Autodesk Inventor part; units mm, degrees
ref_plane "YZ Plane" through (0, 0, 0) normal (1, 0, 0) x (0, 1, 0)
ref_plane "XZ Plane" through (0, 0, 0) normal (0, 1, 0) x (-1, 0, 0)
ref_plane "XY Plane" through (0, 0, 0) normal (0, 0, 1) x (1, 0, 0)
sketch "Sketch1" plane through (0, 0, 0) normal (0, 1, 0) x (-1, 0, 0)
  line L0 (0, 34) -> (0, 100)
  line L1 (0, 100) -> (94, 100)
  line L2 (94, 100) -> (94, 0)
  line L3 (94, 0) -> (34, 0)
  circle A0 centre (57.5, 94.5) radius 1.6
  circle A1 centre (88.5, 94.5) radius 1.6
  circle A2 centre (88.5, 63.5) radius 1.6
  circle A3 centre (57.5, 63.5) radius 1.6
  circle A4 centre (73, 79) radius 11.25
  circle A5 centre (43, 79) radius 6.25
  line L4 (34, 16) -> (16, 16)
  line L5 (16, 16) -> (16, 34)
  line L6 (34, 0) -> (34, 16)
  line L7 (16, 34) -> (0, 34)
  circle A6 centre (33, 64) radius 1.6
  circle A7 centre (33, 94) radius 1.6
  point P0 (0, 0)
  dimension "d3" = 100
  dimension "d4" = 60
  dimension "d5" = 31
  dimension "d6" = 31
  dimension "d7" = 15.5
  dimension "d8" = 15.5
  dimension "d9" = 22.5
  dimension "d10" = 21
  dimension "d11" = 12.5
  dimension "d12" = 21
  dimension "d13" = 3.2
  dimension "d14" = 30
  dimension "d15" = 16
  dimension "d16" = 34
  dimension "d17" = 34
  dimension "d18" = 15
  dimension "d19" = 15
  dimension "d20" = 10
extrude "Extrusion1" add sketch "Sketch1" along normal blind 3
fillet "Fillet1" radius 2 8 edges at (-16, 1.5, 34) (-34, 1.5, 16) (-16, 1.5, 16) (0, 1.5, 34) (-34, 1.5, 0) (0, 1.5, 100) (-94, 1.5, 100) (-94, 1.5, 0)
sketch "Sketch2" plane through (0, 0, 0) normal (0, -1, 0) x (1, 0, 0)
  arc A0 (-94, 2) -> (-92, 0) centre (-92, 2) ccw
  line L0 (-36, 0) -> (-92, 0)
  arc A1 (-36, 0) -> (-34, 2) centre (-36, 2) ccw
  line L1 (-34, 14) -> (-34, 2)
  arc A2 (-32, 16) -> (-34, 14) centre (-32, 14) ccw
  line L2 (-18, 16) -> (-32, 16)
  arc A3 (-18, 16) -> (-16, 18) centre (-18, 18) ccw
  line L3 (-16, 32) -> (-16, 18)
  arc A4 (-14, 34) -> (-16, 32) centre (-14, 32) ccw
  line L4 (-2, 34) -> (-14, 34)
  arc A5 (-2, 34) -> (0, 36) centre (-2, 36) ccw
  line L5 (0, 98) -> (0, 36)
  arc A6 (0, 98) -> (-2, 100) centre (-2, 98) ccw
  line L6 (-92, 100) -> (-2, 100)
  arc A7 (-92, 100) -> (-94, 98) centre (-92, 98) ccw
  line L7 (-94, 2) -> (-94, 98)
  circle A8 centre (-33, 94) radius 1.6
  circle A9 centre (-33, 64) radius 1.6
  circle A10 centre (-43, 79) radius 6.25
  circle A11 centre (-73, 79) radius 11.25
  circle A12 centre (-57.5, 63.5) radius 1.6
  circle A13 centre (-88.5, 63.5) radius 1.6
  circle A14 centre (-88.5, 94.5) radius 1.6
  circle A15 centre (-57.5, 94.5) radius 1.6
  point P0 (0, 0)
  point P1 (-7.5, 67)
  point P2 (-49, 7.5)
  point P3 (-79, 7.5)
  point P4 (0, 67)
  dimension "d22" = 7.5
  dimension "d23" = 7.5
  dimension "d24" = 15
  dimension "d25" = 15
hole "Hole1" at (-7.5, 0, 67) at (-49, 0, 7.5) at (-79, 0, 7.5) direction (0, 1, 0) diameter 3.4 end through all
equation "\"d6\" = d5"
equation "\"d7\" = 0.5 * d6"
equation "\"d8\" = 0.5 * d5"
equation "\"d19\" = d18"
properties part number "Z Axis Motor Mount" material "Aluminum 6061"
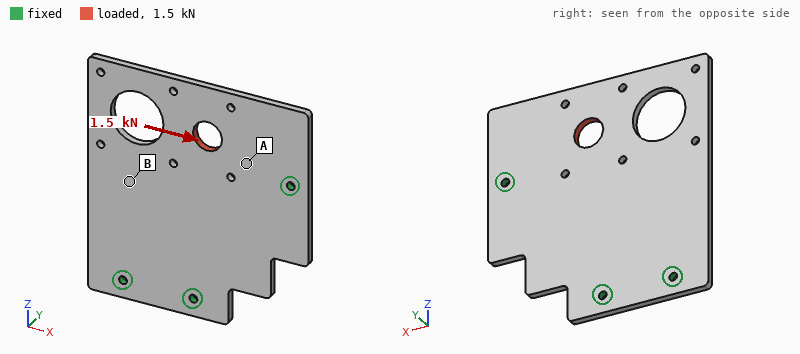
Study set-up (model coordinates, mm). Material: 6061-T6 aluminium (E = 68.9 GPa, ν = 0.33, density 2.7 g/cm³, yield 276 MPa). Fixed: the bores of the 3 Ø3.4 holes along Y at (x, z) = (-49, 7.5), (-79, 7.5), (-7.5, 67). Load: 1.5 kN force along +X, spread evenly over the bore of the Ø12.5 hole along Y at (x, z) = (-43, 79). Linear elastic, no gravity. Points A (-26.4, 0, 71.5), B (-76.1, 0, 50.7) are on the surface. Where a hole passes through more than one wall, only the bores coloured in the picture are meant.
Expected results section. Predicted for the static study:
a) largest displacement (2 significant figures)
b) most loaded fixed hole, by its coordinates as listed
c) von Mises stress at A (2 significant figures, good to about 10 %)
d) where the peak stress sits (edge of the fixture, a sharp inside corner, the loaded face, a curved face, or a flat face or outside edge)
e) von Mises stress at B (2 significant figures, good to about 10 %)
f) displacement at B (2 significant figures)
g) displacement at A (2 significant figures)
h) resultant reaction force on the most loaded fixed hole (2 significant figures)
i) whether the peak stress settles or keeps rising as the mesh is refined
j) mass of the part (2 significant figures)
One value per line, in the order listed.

16 µm
(-7.5, 67)
18 MPa
edge of the fixture
4.1 MPa
6.9 µm
7.0 µm
1.3 kN
keeps rising
65 g
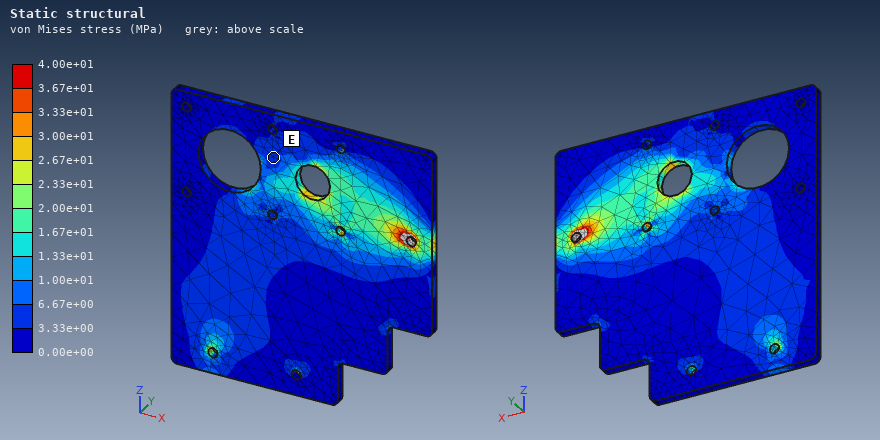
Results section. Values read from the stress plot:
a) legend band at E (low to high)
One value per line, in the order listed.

3.33e+00 to 6.67e+00 MPa
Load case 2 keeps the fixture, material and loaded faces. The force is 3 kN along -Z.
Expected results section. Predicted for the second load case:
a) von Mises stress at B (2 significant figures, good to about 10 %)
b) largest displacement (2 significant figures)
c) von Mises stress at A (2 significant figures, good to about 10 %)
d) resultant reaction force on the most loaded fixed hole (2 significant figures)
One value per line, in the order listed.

9.4 MPa
25 µm
14 MPa
1.1 kN
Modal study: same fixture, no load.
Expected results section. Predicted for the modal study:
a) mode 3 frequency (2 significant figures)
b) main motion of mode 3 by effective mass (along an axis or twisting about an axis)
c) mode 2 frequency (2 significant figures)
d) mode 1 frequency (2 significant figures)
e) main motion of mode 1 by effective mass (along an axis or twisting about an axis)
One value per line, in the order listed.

2000 Hz
along Y
1600 Hz
570 Hz
along Y
